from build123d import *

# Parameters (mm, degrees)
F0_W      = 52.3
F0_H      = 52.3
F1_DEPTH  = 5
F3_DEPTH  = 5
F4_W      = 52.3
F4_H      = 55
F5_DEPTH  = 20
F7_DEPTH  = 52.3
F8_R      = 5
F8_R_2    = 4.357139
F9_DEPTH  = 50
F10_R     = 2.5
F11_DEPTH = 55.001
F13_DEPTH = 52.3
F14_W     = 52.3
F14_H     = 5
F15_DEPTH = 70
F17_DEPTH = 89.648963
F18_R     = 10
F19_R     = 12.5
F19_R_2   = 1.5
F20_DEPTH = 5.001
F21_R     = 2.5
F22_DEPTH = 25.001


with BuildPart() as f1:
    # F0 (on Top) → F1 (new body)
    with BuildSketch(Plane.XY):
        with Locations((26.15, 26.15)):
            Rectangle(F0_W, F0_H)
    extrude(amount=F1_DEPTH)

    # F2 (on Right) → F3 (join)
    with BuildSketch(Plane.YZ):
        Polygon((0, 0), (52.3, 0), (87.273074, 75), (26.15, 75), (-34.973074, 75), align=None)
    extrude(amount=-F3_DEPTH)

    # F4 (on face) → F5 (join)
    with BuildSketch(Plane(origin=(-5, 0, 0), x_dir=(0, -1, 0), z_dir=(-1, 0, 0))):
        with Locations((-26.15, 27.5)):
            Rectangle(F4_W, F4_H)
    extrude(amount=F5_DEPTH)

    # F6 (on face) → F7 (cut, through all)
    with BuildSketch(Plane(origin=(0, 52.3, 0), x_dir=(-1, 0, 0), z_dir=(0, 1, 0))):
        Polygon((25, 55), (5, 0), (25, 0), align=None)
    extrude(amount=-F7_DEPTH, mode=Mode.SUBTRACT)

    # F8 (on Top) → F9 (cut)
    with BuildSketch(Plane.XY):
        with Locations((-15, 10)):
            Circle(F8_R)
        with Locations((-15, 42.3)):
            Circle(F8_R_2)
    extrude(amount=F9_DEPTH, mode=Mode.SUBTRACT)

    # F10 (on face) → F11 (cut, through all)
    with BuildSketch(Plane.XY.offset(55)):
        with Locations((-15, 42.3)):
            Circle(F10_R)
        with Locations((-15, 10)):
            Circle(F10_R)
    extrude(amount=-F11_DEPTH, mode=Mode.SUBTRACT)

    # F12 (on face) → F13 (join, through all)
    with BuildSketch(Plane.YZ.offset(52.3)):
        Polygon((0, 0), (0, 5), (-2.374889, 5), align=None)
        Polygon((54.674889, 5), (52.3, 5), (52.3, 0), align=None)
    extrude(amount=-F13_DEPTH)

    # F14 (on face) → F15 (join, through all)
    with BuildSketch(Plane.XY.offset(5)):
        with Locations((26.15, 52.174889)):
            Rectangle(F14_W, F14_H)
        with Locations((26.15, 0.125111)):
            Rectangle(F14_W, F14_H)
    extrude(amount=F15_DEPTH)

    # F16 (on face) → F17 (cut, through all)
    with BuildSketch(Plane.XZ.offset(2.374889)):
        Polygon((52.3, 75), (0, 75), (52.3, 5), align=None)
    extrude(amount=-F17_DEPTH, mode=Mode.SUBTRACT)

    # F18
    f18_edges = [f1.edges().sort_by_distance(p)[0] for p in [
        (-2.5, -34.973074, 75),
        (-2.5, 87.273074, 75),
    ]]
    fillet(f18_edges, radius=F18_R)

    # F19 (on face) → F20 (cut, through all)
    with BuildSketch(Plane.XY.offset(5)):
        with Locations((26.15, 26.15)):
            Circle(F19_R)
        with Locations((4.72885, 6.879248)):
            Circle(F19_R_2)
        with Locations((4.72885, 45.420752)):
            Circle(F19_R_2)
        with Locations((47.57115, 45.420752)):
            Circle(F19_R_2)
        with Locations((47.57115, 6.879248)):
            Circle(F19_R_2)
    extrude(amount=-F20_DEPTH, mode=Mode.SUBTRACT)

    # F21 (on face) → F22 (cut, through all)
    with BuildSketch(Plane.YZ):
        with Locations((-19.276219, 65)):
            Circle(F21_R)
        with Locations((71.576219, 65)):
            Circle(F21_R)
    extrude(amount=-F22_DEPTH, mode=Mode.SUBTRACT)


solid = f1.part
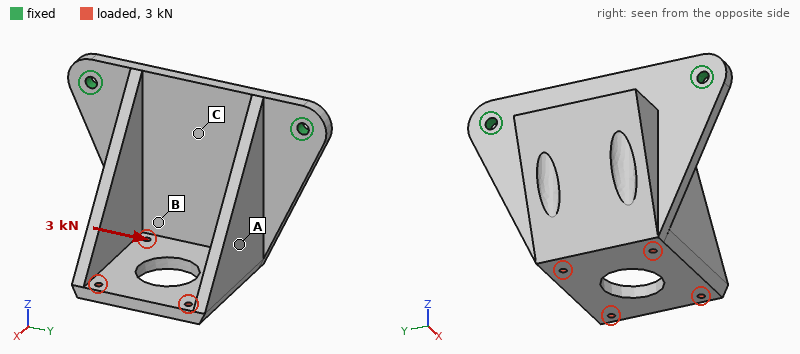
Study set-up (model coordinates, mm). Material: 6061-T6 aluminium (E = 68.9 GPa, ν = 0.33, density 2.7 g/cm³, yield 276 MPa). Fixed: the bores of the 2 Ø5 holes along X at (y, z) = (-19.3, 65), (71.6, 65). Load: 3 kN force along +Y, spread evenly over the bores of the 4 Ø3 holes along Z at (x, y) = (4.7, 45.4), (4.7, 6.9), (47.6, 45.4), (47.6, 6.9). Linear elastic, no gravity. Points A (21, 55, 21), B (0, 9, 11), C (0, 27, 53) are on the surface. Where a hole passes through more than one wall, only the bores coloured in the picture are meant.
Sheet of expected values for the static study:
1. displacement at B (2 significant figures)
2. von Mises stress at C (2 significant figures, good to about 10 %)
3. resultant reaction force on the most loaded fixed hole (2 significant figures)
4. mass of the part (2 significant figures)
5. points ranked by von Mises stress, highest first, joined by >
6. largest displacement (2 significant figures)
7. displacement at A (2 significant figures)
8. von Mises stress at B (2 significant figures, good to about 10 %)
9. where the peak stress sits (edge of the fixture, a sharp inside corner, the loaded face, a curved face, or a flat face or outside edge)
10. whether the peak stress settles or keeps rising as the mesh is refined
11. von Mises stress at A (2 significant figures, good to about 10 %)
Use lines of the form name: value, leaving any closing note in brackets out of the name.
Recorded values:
displacement at B: 0.099 mm
von Mises stress at C: 27 MPa
resultant reaction force on the most loaded fixed hole: 2.8 kN
mass of the part: 240 g
points ranked by von Mises stress, highest first, joined by >: B > C > A
largest displacement: 0.45 mm
displacement at A: 0.22 mm
von Mises stress at B: 39 MPa
where the peak stress sits: edge of the fixture
whether the peak stress settles or keeps rising as the mesh is refined: keeps rising
von Mises stress at A: 21 MPa
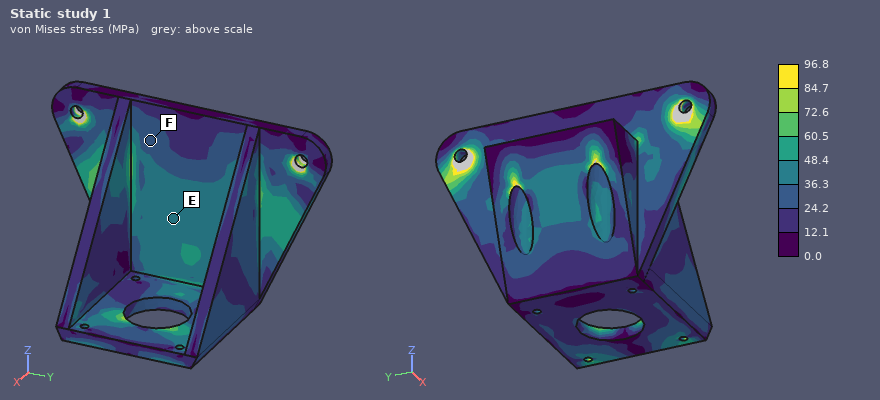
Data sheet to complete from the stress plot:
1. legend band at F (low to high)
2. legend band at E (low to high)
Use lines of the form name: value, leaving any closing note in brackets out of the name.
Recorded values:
legend band at F: 24.2 to 36.3 MPa
legend band at E: 36.3 to 48.4 MPa
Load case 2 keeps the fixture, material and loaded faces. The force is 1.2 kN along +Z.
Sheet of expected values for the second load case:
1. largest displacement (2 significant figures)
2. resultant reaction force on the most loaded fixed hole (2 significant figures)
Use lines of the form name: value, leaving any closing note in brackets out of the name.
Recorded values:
largest displacement: 0.82 mm
resultant reaction force on the most loaded fixed hole: 640 N
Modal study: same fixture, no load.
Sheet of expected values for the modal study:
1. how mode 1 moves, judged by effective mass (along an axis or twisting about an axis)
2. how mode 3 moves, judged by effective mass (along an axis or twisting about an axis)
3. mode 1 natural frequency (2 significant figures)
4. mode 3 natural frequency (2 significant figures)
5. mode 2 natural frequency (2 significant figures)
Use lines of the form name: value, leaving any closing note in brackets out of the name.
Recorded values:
how mode 1 moves, judged by effective mass: along X
how mode 3 moves, judged by effective mass: along X
mode 1 natural frequency: 490 Hz
mode 3 natural frequency: 2900 Hz
mode 2 natural frequency: 1800 Hz
